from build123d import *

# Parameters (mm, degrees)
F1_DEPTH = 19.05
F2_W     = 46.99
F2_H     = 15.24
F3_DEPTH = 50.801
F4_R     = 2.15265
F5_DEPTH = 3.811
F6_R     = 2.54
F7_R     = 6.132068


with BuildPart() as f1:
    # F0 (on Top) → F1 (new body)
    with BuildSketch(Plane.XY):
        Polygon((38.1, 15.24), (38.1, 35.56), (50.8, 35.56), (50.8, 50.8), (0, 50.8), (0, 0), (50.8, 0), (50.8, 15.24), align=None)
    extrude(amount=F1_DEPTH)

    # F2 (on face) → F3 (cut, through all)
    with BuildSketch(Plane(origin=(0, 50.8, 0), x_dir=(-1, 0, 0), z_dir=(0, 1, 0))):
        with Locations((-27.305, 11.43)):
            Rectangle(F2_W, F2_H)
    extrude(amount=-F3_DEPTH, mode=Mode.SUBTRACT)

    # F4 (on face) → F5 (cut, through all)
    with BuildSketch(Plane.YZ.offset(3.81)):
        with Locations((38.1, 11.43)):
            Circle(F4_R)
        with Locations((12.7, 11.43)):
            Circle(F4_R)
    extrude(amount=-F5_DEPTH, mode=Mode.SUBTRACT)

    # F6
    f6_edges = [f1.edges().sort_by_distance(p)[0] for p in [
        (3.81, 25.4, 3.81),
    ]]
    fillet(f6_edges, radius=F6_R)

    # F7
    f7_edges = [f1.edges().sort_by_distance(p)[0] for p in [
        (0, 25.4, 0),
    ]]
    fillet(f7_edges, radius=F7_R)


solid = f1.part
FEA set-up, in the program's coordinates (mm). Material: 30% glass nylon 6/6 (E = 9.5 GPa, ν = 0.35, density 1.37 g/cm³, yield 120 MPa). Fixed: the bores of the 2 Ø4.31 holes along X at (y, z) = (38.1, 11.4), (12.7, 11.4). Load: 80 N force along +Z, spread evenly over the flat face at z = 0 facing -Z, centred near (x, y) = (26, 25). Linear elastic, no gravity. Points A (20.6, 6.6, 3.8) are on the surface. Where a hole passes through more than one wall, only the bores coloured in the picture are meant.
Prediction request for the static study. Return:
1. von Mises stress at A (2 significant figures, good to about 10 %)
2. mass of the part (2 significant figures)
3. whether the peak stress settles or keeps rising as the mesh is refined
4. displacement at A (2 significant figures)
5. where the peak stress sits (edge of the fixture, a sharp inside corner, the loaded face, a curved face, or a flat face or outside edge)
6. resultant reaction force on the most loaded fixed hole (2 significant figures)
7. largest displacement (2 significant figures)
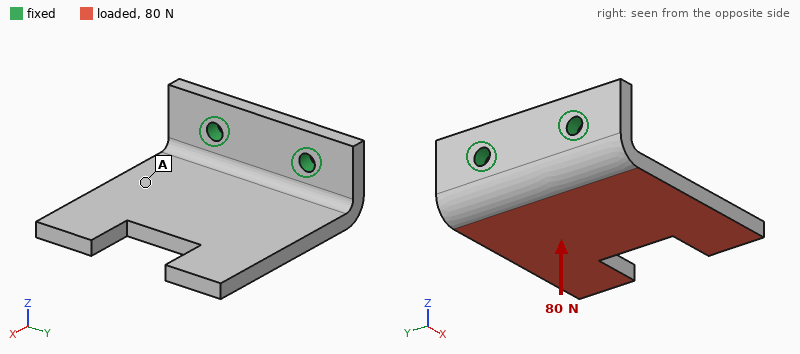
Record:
5.3 MPa
16 g
keeps rising
0.23 mm
edge of the fixture
41 N
0.80 mm
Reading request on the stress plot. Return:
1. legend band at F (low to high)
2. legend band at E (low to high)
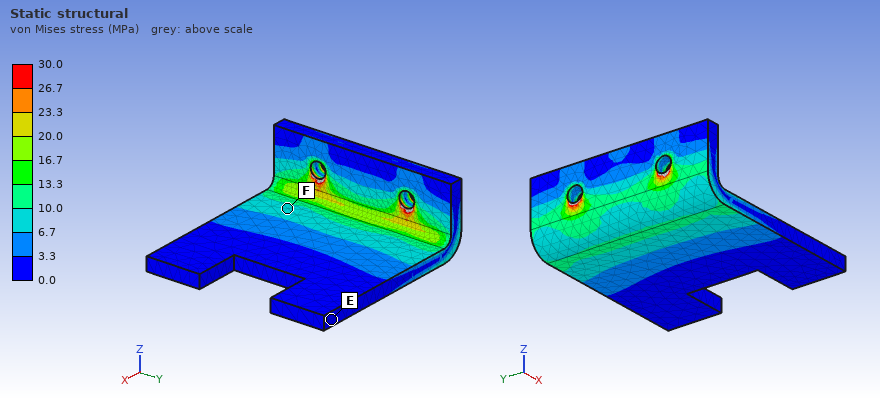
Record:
6.7 to 10.0 MPa
0.0 to 3.3 MPa
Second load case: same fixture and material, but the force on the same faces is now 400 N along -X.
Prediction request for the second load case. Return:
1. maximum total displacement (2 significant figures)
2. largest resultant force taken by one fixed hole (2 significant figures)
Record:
0.84 mm
200 N
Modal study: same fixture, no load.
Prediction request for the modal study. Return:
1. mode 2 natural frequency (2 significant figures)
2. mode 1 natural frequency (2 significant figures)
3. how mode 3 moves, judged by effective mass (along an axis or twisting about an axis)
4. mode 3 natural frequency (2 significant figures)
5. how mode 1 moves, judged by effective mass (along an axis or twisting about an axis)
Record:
1200 Hz
630 Hz
along Y
2200 Hz
along Z
